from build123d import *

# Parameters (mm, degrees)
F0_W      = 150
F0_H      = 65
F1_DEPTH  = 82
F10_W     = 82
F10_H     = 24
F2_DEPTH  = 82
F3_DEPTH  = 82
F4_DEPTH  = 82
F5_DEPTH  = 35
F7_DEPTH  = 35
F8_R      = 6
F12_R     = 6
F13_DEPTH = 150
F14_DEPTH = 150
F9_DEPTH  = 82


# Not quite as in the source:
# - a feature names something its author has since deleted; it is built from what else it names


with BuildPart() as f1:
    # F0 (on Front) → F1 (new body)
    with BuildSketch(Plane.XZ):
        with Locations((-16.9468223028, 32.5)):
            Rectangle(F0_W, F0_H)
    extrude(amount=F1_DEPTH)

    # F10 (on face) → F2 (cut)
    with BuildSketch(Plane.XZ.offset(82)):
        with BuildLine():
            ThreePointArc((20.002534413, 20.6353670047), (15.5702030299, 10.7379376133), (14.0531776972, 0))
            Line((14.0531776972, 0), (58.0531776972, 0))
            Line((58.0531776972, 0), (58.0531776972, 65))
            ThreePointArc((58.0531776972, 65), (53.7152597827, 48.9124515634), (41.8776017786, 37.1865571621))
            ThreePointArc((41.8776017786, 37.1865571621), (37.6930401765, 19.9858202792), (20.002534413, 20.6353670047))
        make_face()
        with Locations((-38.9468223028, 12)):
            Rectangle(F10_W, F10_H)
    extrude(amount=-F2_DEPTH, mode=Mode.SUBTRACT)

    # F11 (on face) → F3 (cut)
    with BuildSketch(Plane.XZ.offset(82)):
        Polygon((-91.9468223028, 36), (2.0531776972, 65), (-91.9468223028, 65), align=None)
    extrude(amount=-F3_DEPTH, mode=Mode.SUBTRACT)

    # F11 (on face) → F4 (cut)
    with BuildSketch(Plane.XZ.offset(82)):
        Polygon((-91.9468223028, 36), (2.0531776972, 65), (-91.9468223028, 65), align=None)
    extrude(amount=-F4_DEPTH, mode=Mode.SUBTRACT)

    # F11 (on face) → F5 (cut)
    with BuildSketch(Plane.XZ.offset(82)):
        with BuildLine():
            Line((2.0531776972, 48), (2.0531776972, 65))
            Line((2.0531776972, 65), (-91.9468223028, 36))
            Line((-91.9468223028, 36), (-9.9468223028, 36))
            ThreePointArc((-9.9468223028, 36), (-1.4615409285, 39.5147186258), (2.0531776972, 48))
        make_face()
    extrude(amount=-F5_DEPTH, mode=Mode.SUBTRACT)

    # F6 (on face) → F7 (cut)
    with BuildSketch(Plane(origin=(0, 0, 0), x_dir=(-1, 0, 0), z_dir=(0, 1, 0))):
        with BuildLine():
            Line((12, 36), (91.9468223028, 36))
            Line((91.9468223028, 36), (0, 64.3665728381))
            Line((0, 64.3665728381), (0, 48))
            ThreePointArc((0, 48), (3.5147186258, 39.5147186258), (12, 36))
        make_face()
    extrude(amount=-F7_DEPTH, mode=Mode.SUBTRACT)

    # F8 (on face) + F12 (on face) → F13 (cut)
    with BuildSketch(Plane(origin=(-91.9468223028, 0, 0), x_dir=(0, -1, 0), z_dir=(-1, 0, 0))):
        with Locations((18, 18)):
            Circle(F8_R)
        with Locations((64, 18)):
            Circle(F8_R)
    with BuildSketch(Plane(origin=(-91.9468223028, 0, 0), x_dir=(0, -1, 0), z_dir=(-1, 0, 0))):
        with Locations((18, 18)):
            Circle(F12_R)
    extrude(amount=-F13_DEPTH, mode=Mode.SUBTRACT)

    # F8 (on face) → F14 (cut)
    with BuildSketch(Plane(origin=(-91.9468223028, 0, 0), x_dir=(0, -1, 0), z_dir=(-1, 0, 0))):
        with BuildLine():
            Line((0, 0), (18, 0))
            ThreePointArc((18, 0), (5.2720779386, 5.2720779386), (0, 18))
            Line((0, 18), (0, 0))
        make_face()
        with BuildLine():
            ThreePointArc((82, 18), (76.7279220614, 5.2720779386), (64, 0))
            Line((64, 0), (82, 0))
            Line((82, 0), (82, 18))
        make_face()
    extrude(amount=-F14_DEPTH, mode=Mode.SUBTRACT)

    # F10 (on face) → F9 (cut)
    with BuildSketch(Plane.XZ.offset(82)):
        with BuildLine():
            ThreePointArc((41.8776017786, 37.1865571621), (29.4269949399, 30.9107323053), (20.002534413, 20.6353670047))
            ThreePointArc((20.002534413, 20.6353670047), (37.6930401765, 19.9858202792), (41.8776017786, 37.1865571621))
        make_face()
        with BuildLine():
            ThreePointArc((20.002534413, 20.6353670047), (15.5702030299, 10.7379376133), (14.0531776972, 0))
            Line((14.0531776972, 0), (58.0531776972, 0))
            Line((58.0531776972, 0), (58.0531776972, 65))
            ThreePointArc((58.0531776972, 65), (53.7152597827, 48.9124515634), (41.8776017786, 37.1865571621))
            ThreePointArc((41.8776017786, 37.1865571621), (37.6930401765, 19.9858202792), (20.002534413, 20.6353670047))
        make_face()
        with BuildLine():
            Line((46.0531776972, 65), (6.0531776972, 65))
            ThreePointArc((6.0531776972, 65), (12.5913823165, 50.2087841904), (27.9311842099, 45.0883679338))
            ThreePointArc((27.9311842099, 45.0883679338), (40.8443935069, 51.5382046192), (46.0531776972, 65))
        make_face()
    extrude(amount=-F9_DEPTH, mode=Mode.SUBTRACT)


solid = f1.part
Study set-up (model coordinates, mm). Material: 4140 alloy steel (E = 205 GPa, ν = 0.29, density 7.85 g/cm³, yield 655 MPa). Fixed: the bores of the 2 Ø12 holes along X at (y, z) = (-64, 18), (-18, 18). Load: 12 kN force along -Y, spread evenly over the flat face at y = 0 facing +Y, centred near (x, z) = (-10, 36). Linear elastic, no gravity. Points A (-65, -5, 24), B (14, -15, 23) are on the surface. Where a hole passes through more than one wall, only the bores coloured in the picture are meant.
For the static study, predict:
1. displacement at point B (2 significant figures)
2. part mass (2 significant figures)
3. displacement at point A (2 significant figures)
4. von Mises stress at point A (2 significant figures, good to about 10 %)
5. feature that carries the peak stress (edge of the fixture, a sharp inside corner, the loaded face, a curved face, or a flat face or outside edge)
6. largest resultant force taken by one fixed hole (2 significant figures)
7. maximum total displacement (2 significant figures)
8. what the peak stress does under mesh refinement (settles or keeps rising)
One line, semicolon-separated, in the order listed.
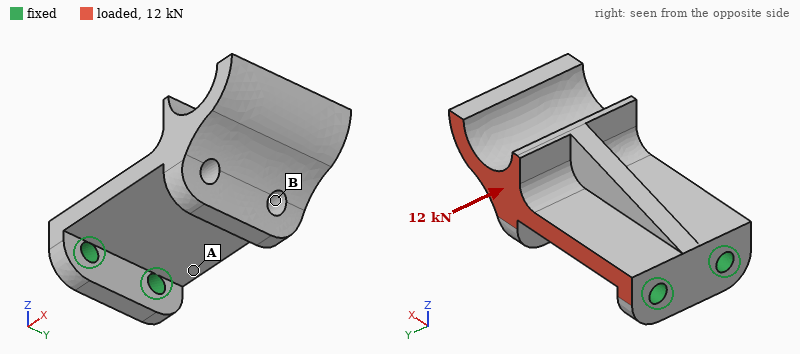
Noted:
0.064 mm; 2.0 kg; 0.021 mm; 69 MPa; edge of the fixture; 18 kN; 0.11 mm; keeps rising
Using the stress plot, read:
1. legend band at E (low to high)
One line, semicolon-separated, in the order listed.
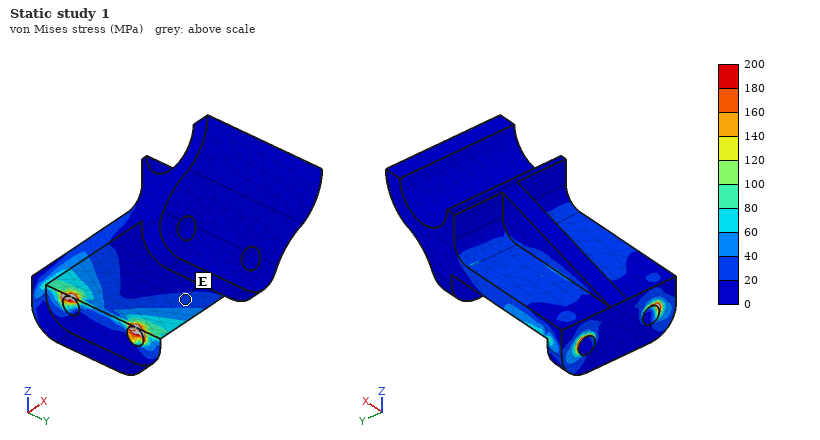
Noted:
20 to 40 MPa
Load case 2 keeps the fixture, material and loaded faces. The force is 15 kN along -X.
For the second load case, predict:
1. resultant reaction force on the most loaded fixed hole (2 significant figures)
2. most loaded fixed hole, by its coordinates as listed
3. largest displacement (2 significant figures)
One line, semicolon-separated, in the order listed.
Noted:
19 kN; (-18, 18); 0.30 mm
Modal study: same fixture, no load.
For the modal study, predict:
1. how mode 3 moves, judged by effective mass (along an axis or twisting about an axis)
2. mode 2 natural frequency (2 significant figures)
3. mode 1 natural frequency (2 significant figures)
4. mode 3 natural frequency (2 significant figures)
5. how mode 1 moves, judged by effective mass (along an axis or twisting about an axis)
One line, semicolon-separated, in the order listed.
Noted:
along Y; 1400 Hz; 400 Hz; 1600 Hz; along Z
